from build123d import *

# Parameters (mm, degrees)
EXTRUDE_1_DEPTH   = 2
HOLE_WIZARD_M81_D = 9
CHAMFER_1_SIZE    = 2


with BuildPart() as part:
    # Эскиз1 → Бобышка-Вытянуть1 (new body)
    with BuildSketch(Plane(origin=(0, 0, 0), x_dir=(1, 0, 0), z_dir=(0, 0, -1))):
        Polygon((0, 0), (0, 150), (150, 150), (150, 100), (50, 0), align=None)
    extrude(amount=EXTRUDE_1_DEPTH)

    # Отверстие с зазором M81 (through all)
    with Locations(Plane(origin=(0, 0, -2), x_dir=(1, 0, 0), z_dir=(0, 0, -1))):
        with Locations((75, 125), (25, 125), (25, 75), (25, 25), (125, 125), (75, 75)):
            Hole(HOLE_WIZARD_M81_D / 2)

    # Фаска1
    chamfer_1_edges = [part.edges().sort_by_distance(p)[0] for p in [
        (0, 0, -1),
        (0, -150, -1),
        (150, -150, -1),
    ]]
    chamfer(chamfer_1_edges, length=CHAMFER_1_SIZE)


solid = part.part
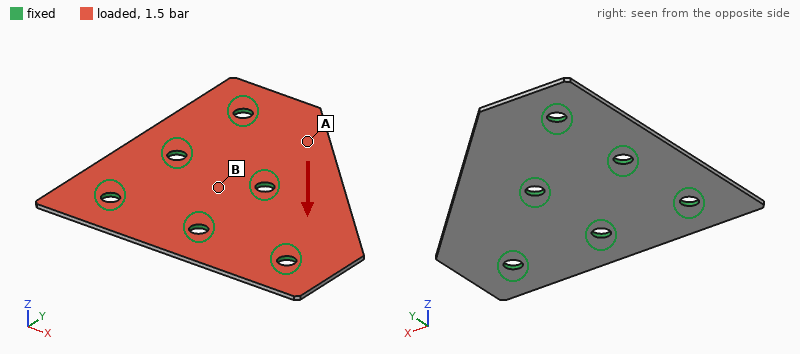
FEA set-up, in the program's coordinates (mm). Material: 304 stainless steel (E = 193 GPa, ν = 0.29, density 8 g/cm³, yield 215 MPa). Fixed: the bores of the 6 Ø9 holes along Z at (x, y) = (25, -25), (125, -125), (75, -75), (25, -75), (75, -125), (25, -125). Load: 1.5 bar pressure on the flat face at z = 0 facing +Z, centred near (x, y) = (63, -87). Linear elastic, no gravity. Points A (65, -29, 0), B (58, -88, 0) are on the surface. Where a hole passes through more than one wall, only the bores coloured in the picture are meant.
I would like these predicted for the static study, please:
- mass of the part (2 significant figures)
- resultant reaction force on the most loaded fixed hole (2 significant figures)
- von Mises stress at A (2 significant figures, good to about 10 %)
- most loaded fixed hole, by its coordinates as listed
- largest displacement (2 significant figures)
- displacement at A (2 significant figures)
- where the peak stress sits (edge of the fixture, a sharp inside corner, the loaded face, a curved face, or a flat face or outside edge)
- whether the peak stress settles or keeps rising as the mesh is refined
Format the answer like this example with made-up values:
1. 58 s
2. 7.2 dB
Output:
1. 270 g
2. 600 N
3. 39 MPa
4. (75, -75)
5. 0.27 mm
6. 0.19 mm
7. edge of the fixture
8. keeps rising
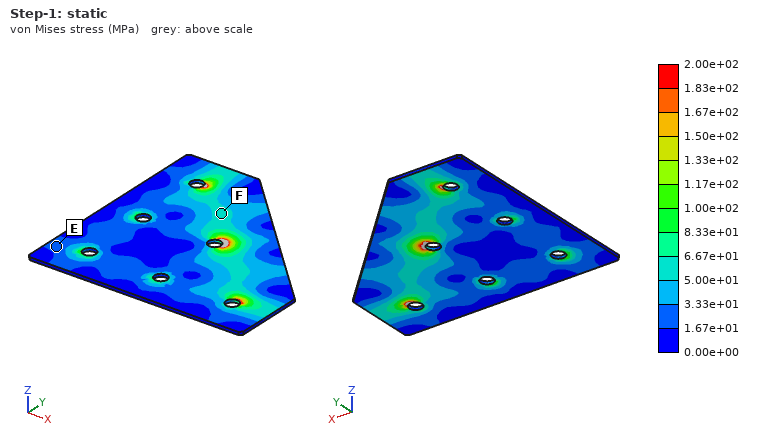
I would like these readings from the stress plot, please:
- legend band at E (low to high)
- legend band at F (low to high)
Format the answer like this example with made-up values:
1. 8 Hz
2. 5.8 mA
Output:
1. 1.67e+01 to 3.33e+01 MPa
2. 5.00e+01 to 6.67e+01 MPa
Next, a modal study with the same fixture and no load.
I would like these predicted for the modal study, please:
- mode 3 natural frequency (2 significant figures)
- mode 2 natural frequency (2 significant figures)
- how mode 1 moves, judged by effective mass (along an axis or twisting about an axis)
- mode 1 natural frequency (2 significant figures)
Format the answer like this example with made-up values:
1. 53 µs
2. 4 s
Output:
1. 2300 Hz
2. 1400 Hz
3. along Z
4. 1200 Hz
